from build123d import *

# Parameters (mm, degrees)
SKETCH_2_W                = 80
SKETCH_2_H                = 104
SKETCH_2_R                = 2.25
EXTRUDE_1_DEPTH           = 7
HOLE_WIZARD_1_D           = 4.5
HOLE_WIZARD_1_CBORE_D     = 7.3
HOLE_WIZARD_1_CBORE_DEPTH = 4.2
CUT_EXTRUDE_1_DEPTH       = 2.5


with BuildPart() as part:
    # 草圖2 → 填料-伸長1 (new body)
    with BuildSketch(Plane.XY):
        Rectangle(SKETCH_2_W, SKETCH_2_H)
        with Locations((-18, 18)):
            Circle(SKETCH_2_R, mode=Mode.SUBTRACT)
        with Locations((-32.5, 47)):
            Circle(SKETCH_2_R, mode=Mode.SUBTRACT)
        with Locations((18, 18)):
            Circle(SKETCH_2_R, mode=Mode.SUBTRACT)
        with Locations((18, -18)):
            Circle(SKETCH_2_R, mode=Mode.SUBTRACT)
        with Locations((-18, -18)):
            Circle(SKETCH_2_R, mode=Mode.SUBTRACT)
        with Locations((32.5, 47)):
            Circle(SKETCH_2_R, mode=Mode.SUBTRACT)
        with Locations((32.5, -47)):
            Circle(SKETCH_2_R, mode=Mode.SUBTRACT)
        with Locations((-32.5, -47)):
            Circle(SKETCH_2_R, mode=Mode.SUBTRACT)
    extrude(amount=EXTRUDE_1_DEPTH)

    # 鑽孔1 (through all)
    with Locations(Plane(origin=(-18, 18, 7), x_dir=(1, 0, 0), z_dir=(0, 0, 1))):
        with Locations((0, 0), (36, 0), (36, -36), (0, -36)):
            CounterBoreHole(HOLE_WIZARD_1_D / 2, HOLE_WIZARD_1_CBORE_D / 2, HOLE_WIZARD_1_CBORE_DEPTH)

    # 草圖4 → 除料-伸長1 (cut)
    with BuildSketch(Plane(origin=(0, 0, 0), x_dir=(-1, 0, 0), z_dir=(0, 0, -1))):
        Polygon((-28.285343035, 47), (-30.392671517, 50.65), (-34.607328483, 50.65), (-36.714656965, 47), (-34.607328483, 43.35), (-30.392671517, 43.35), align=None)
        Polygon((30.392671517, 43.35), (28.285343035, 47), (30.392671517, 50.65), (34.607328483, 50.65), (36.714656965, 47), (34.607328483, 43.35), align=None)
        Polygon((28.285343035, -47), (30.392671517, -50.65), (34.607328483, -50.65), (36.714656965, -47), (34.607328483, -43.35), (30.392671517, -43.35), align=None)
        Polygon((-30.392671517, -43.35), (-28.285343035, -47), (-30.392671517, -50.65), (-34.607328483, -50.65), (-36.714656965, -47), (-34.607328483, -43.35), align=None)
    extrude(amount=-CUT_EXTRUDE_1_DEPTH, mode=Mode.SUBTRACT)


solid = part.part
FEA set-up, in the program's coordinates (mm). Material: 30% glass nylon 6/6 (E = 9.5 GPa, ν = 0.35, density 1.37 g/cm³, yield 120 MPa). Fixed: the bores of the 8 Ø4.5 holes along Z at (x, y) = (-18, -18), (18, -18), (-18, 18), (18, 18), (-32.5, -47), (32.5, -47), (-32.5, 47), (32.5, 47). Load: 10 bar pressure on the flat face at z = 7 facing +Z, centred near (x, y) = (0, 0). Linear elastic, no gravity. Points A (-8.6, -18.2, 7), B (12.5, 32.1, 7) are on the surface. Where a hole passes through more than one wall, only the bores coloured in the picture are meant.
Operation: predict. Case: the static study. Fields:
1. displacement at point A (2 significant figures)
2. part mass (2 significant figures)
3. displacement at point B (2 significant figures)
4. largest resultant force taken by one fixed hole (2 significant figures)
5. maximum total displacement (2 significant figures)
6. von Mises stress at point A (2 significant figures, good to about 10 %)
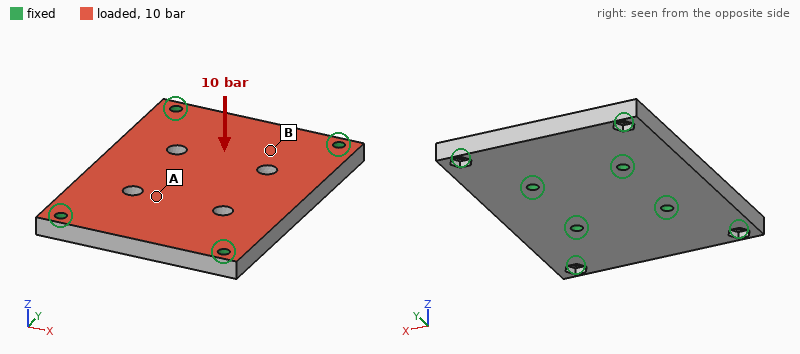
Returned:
0.039 mm
78 g
0.076 mm
1.3 kN
0.18 mm
14 MPa
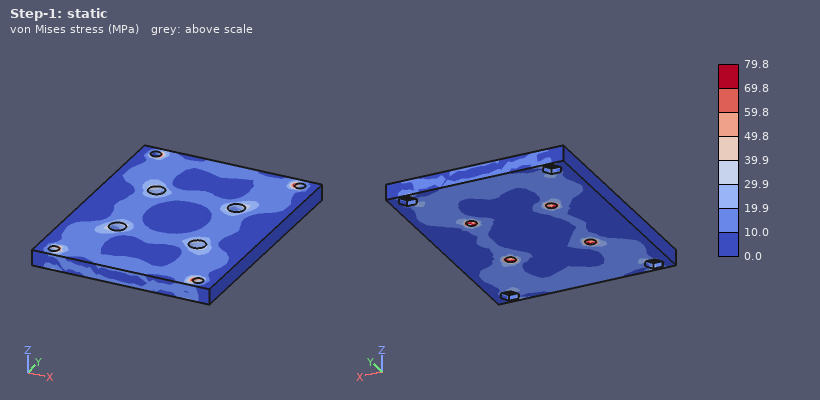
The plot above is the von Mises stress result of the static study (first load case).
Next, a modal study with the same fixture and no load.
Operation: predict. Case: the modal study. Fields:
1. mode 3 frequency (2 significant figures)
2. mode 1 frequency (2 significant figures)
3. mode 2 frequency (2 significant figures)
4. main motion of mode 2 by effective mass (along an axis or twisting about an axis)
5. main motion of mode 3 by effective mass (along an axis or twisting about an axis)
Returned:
4700 Hz
4000 Hz
4500 Hz
twisting about X
twisting about Y
